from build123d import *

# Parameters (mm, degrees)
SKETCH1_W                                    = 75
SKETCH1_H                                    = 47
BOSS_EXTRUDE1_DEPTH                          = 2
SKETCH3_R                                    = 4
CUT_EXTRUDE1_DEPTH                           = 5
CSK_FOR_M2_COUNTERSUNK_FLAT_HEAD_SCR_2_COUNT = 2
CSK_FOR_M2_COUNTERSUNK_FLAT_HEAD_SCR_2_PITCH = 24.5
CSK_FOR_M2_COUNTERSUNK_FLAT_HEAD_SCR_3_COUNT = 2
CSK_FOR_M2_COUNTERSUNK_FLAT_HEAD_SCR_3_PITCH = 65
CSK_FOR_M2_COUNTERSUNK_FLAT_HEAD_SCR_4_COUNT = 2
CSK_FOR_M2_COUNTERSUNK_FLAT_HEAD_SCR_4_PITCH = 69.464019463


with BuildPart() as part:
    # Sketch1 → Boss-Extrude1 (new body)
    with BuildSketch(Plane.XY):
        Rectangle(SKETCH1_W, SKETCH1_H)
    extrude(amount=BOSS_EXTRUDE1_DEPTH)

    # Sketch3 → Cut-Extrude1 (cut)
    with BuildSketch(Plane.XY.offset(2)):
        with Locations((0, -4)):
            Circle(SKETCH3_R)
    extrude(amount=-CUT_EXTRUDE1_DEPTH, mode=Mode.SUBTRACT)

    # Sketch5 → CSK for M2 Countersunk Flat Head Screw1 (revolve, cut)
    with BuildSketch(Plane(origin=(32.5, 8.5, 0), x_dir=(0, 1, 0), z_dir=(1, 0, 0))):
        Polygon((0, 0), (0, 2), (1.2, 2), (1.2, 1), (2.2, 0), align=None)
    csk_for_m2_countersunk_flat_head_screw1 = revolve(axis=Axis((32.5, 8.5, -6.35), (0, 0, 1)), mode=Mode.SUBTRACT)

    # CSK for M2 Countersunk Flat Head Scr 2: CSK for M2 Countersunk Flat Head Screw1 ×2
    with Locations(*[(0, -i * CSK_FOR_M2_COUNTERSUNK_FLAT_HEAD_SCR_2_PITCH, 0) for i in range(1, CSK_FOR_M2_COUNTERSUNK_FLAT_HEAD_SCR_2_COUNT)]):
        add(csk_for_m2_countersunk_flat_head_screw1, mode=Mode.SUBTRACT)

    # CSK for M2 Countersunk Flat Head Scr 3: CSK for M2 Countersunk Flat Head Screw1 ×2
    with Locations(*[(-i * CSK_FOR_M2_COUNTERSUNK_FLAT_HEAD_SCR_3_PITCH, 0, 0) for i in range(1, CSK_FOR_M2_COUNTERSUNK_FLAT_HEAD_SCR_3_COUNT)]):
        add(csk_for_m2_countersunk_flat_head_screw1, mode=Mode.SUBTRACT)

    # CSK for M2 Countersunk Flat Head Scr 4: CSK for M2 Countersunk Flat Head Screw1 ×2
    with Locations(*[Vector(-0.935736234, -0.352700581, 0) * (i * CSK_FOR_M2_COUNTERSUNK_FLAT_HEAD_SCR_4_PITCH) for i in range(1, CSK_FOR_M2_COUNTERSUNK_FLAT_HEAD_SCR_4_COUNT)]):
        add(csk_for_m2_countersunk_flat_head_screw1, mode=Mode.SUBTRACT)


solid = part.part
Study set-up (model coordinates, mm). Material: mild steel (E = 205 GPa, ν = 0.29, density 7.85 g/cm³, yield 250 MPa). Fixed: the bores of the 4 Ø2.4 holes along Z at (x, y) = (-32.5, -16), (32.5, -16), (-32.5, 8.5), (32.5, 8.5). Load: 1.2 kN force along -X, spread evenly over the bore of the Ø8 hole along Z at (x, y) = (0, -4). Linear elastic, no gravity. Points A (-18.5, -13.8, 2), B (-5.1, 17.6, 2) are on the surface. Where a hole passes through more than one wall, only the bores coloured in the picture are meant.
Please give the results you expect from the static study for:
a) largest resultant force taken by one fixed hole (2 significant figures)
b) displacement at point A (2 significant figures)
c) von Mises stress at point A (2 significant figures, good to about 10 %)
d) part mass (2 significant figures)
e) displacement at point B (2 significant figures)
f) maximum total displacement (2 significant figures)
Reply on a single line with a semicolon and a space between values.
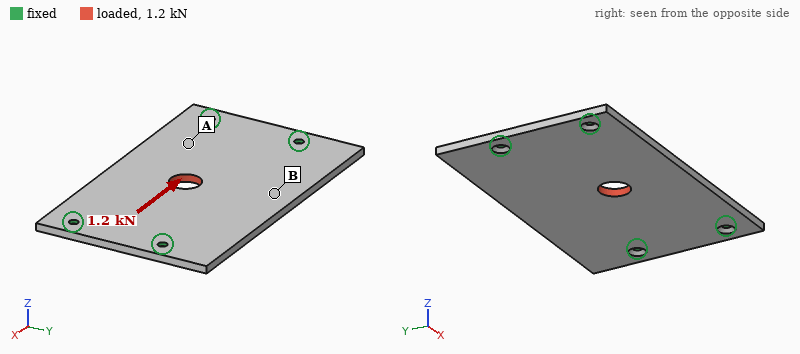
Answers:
300 N; 1.5 µm; 11 MPa; 54 g; 1.0 µm; 2.4 µm
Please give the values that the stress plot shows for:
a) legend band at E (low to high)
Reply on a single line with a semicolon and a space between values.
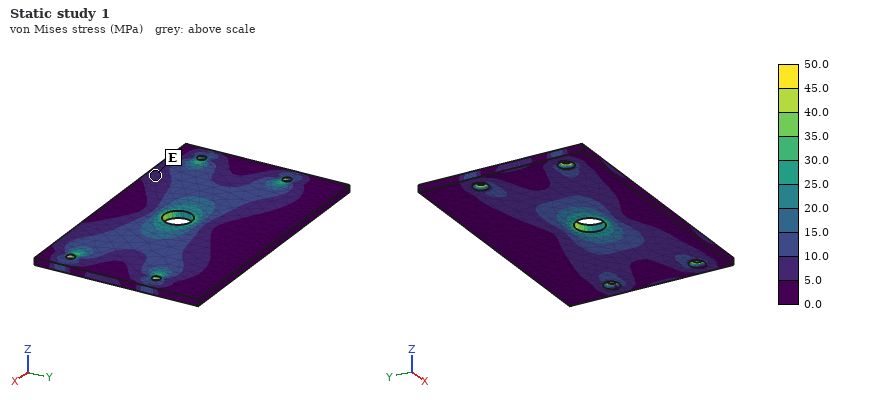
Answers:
5.0 to 10.0 MPa
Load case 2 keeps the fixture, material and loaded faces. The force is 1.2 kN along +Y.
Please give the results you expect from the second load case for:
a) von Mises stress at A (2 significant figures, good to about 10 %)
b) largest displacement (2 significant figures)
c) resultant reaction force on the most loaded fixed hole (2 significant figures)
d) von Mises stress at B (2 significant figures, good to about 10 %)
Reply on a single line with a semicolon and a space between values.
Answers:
13 MPa; 5.1 µm; 370 N; 13 MPa
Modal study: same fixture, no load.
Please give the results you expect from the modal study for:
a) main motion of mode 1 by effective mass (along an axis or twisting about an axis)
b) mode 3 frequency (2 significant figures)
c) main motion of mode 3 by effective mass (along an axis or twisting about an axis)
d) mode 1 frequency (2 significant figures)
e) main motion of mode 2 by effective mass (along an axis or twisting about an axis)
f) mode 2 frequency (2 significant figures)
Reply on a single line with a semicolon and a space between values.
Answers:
along Z; 5000 Hz; twisting about Y; 1900 Hz; twisting about X; 2700 Hz
